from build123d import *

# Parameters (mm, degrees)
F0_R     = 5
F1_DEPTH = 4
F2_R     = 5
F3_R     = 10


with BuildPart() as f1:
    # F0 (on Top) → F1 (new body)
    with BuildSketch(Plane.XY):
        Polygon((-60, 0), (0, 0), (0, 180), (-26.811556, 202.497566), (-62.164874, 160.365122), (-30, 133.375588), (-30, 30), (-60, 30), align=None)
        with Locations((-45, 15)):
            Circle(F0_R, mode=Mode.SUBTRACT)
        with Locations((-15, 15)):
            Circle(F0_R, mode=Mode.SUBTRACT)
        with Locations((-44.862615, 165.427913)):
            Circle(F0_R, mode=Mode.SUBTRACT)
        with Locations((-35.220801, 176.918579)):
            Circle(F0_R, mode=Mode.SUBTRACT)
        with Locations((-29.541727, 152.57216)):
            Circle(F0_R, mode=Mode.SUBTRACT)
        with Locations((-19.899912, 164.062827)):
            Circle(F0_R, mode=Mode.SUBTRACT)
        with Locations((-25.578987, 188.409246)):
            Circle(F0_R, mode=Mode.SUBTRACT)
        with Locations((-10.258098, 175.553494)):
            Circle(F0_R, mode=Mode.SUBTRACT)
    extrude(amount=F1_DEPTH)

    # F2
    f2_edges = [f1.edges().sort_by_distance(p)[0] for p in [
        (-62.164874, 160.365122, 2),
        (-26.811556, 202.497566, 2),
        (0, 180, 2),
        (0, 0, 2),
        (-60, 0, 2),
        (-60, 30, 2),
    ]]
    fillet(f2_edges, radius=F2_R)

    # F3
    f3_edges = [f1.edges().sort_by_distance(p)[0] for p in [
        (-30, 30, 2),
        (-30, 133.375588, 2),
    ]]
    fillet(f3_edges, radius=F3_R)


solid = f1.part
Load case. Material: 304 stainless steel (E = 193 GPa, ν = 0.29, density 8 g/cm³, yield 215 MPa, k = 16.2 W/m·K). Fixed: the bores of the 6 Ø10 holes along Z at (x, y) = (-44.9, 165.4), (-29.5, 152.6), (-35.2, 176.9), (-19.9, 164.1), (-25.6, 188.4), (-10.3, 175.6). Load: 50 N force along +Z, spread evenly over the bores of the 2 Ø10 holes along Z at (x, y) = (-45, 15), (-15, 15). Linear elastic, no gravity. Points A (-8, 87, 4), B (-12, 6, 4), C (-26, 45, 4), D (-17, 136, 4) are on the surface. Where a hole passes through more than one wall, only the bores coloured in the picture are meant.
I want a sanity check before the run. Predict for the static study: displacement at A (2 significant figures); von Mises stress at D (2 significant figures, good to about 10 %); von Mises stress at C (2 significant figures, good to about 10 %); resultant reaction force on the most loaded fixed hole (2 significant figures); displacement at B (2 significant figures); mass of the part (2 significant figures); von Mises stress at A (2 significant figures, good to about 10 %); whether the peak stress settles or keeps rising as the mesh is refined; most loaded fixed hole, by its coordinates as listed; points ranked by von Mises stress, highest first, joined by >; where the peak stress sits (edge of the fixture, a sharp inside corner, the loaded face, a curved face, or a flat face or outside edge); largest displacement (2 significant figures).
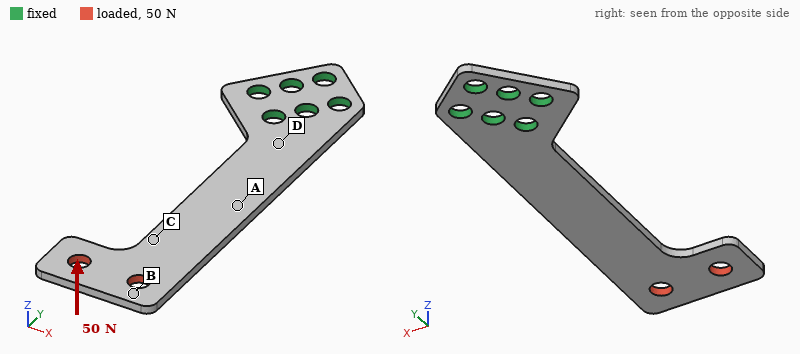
0.36 mm
66 MPa
23 MPa
250 N
1.4 mm
230 g
45 MPa
keeps rising
(-29.5, 152.6)
D > A > C > B
edge of the fixture
1.6 mm
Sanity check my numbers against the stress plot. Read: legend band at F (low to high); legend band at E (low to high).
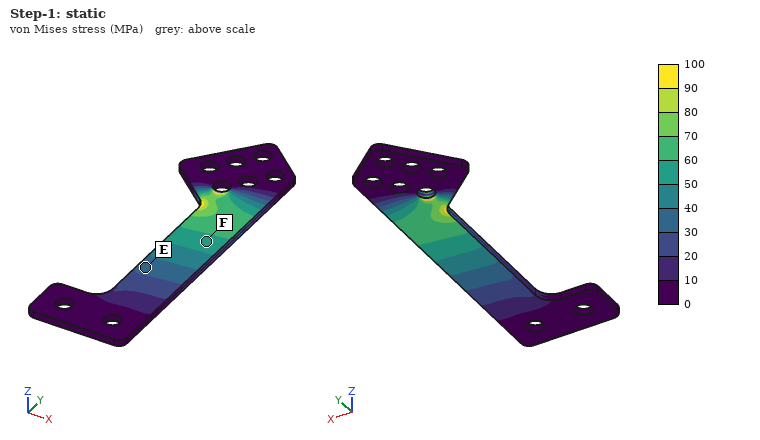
50 to 60 MPa
30 to 40 MPa
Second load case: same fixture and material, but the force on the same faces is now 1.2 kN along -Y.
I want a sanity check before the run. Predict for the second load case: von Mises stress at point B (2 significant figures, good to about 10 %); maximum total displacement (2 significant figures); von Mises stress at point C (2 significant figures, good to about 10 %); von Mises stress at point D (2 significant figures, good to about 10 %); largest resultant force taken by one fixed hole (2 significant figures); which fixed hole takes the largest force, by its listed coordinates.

5.4 MPa
0.12 mm
33 MPa
11 MPa
960 N
(-29.5, 152.6)
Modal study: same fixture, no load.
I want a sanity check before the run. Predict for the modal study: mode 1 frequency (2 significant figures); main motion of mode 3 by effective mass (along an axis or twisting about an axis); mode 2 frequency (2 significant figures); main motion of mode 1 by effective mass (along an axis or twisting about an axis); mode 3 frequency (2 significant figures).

120 Hz
along X
580 Hz
along Z
850 Hz
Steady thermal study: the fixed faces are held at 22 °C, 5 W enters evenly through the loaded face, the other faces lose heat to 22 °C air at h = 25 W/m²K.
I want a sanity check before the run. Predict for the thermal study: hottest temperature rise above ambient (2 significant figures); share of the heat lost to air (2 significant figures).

44 K
98 %
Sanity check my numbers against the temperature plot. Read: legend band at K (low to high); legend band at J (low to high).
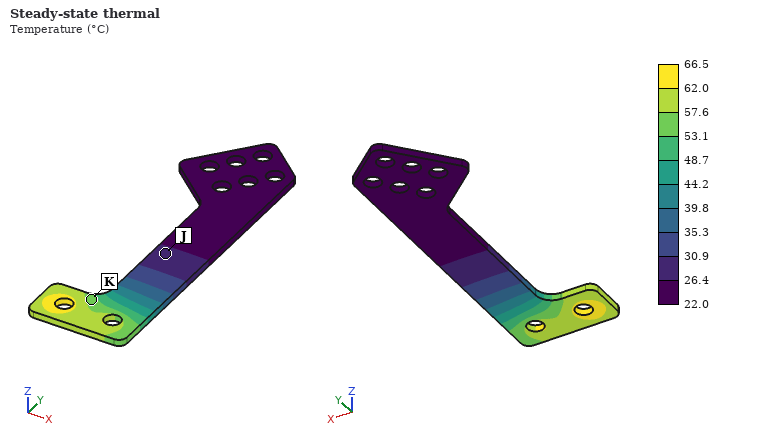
53.1 to 57.6 °C
26.4 to 30.9 °C
